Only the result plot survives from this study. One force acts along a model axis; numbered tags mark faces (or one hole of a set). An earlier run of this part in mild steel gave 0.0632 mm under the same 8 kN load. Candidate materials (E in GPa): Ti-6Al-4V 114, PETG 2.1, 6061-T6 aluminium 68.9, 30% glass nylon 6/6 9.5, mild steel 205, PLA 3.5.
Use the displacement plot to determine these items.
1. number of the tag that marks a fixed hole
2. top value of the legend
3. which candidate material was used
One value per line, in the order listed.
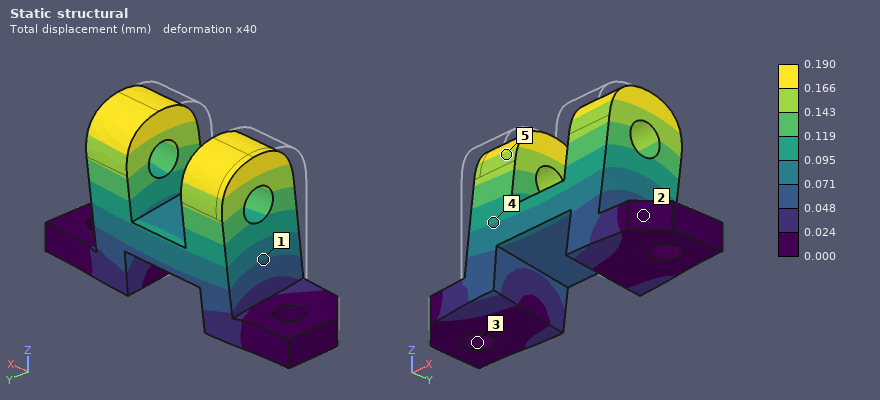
3
0.190 mm
6061-T6 aluminium
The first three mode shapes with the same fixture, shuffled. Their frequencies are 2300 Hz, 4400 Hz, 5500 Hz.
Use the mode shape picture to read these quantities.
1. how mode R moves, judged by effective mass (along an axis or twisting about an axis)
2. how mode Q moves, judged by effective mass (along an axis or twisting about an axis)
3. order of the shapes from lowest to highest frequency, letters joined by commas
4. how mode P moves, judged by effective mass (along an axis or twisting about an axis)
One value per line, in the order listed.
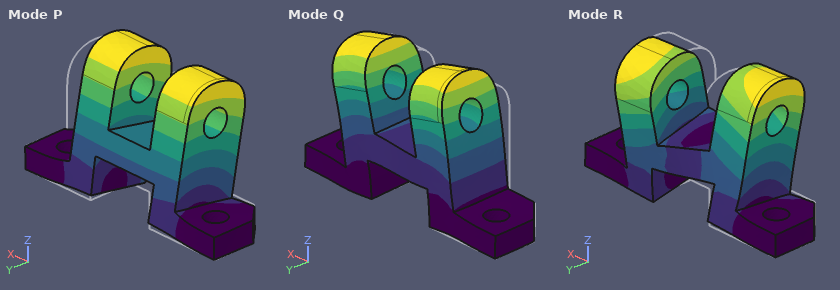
twisting about Z
along X
P, R, Q
along Y
